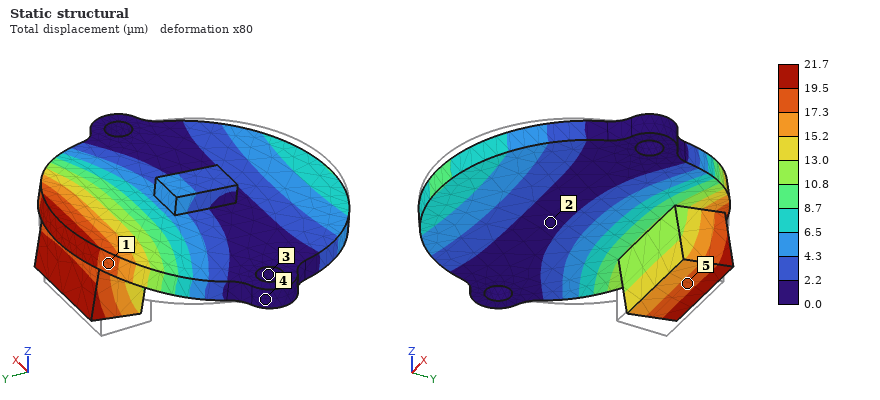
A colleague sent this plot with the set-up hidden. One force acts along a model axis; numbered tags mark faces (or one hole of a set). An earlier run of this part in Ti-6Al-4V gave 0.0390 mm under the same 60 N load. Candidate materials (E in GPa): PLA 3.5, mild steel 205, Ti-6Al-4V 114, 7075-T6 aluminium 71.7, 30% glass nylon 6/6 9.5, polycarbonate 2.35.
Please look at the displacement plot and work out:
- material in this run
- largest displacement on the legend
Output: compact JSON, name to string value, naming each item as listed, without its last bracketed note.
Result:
{"material in this run": "mild steel", "largest displacement on the legend": "21.7 µm"}
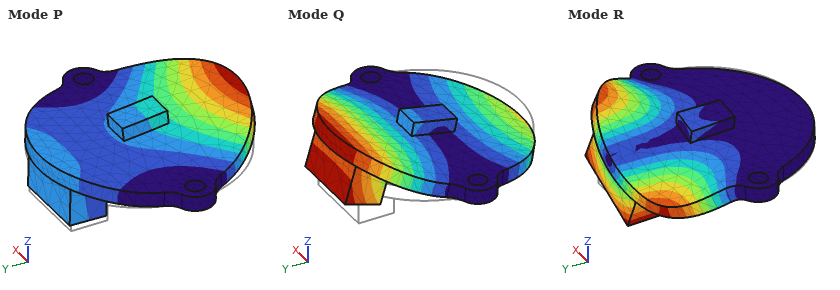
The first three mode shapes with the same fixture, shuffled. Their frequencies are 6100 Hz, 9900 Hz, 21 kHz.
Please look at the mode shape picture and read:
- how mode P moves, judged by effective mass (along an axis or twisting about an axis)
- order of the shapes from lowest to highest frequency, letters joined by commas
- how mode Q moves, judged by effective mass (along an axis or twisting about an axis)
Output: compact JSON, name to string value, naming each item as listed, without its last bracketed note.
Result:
{"how mode P moves, judged by effective mass": "along Z", "order of the shapes from lowest to highest frequency, letters joined by commas": "Q, P, R", "how mode Q moves, judged by effective mass": "along Z"}
